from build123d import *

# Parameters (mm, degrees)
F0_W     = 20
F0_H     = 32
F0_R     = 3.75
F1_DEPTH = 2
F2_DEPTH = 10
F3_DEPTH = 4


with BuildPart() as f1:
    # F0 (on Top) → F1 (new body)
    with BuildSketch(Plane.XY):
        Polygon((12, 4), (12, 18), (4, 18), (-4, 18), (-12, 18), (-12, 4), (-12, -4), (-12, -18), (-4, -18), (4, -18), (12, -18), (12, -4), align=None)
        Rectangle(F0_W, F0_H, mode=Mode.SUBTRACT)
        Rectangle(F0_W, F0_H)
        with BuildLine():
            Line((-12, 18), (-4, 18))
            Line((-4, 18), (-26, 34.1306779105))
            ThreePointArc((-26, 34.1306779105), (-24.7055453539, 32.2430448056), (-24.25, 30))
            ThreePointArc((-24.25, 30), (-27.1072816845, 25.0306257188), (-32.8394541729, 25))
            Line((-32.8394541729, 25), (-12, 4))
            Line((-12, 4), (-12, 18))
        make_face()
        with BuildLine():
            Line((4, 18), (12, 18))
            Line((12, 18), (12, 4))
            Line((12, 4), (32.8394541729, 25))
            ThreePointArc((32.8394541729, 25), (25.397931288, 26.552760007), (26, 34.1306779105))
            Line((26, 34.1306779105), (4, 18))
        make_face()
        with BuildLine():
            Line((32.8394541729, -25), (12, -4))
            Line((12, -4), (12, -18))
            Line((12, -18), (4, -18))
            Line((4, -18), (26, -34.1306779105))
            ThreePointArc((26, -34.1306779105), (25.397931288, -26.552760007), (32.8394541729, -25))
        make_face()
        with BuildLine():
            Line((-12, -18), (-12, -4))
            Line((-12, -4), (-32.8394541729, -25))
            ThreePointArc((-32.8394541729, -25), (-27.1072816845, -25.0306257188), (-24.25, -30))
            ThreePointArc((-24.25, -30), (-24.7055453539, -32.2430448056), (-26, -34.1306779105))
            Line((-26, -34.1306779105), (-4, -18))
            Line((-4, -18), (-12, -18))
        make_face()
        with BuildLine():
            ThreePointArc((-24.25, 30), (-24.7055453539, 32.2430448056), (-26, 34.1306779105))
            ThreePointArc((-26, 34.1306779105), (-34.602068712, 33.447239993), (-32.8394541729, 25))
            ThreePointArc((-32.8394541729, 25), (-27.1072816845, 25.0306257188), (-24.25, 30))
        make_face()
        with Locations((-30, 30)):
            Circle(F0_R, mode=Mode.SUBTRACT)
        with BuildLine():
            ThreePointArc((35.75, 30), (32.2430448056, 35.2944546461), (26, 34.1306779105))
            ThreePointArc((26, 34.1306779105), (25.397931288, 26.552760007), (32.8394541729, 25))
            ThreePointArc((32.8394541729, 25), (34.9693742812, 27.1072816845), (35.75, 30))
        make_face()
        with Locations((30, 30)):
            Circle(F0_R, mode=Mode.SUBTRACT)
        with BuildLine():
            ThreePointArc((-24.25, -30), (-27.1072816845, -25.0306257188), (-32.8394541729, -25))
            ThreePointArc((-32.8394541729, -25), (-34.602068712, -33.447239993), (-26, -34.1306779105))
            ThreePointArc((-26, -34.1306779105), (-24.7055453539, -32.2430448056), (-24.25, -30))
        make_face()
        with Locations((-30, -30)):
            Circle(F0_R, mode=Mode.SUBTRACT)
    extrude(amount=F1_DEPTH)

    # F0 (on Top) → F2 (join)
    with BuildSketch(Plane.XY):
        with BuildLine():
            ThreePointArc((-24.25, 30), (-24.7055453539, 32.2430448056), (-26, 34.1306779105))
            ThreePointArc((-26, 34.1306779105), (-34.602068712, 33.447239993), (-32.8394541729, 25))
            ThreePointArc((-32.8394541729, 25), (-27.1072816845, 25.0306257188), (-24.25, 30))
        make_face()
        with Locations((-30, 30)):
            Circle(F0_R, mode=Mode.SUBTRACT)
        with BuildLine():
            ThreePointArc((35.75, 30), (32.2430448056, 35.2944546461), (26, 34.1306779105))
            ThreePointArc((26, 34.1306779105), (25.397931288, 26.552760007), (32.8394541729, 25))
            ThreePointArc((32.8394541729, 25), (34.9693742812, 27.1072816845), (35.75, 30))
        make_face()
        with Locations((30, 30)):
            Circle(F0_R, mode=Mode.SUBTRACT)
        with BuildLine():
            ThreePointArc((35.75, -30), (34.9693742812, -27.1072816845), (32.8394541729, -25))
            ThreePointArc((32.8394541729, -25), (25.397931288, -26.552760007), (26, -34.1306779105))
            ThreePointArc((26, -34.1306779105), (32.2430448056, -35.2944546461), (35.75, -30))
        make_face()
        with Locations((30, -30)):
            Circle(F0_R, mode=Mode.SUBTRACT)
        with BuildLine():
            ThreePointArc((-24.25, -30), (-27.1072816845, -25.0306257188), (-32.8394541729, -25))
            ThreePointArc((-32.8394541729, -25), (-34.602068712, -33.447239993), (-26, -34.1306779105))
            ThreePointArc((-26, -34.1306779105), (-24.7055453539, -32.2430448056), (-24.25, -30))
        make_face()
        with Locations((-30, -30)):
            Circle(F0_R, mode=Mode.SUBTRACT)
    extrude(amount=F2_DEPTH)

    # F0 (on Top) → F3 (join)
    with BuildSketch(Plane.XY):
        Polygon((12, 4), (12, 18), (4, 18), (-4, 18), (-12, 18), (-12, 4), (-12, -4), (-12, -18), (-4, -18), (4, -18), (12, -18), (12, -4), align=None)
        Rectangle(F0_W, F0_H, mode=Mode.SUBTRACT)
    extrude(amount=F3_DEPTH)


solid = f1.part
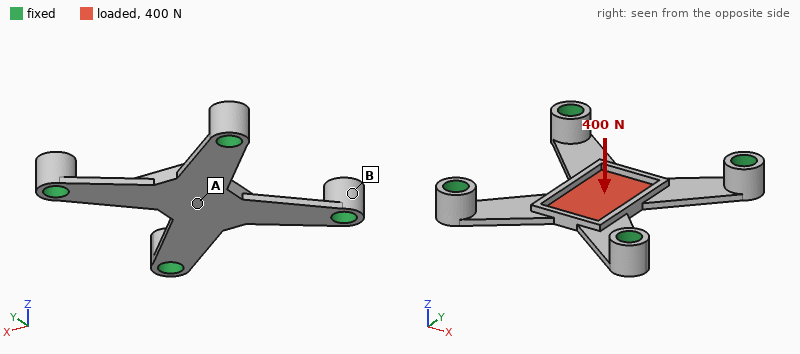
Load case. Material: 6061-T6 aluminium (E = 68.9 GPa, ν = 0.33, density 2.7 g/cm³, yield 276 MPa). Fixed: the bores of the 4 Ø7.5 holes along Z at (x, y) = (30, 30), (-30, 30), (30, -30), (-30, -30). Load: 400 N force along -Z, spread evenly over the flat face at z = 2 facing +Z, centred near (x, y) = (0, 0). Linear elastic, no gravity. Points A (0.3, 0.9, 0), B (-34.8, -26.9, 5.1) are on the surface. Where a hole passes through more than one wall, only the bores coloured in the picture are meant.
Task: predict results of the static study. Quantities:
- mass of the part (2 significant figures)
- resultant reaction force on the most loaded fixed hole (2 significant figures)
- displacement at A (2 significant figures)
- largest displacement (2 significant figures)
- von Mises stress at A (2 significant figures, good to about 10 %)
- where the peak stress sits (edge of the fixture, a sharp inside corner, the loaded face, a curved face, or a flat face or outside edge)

18 g
140 N
0.28 mm
0.28 mm
65 MPa
a flat face or outside edge
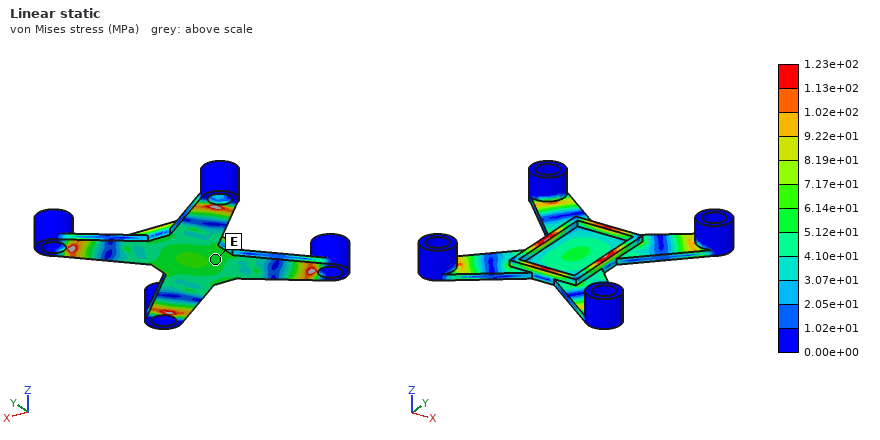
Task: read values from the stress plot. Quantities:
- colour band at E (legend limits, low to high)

5.12e+01 to 6.14e+01 MPa
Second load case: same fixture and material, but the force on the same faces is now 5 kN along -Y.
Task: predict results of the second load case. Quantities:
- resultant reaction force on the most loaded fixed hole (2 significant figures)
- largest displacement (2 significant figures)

1.7 kN
0.10 mm
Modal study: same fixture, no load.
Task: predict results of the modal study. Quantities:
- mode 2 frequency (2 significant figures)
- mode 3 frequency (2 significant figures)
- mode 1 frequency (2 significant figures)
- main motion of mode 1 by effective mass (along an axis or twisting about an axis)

5000 Hz
5600 Hz
2500 Hz
along Z
